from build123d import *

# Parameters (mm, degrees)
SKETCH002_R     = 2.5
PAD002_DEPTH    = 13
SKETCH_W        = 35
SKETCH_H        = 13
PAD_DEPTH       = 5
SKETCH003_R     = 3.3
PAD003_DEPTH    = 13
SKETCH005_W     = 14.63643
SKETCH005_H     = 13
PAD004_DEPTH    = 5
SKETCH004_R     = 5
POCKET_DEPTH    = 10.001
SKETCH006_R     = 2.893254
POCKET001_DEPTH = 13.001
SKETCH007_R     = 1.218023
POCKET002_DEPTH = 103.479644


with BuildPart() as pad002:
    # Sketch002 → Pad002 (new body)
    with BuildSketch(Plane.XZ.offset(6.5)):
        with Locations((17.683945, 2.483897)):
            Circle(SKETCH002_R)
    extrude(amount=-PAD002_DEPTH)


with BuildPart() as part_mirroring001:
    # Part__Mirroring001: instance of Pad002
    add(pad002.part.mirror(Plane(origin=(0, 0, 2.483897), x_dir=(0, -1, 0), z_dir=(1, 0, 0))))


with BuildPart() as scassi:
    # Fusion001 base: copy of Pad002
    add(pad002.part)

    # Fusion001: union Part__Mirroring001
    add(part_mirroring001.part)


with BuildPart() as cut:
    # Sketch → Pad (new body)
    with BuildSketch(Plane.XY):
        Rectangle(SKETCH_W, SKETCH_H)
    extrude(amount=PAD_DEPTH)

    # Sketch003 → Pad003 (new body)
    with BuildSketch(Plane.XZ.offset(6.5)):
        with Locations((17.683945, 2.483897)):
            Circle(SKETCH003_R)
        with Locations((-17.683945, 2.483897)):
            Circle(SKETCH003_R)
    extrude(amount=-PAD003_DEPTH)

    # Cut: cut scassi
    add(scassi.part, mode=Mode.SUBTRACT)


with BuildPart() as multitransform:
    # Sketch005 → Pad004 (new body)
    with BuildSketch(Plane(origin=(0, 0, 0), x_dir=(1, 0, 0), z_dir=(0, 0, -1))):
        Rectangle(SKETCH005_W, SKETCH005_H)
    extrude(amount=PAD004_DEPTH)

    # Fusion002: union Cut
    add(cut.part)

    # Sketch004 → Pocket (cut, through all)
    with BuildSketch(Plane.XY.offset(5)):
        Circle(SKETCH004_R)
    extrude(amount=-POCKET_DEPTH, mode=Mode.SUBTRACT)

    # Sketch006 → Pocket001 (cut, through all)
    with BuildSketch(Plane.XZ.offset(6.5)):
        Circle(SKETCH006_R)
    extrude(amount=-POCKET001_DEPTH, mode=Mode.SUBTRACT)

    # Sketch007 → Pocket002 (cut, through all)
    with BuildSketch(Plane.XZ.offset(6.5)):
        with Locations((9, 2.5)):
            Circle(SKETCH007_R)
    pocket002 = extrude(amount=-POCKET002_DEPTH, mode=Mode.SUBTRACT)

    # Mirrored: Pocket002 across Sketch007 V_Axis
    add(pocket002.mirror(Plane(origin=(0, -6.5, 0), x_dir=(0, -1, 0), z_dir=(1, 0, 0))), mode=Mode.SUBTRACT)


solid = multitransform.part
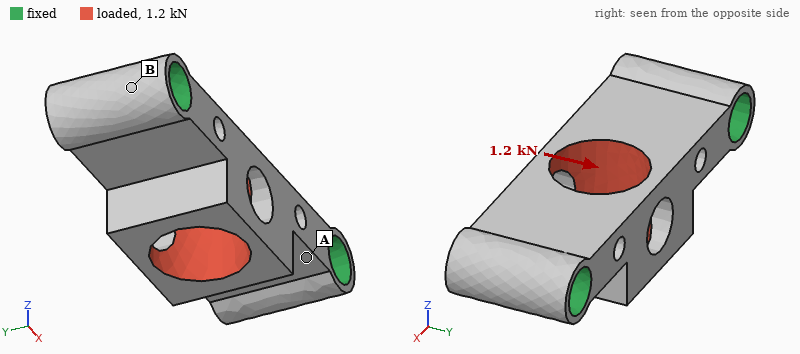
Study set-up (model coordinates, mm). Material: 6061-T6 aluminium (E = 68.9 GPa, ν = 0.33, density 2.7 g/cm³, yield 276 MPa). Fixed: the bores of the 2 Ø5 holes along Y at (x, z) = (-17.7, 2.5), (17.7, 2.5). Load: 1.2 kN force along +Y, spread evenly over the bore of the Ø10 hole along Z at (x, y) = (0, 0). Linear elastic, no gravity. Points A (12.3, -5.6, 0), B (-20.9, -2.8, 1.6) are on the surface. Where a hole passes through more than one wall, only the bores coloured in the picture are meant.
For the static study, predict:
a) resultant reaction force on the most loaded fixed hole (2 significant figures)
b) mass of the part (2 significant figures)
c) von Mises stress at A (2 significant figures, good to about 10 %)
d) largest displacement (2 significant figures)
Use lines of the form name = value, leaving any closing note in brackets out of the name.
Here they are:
resultant reaction force on the most loaded fixed hole = 600 N
mass of the part = 6.1 g
von Mises stress at A = 24 MPa
largest displacement = 22 µm
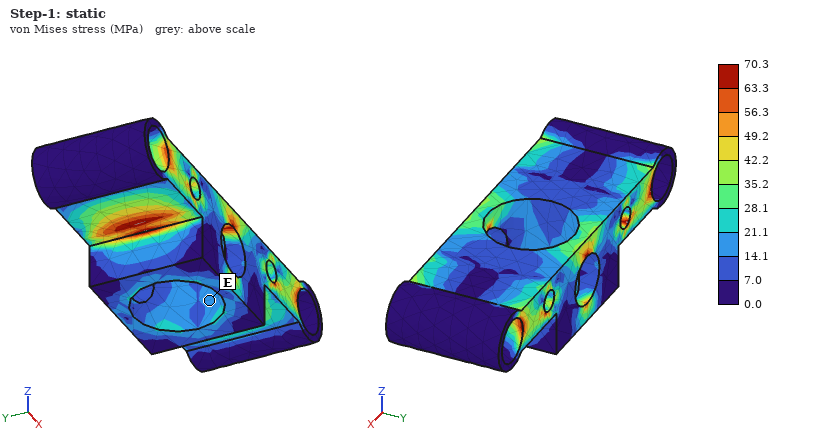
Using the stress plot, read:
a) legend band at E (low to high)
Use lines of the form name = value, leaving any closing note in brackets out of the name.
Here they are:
legend band at E = 14.1 to 21.1 MPa
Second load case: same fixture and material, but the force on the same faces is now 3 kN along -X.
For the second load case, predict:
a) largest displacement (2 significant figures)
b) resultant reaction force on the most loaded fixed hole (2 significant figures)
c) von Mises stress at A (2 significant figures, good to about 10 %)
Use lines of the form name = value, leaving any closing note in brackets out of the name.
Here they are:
largest displacement = 17 µm
resultant reaction force on the most loaded fixed hole = 1.5 kN
von Mises stress at A = 35 MPa
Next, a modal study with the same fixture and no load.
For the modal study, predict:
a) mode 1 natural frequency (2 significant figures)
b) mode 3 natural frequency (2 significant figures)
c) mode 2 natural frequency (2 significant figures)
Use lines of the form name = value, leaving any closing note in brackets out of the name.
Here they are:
mode 1 natural frequency = 23 kHz
mode 3 natural frequency = 37 kHz
mode 2 natural frequency = 23 kHz
